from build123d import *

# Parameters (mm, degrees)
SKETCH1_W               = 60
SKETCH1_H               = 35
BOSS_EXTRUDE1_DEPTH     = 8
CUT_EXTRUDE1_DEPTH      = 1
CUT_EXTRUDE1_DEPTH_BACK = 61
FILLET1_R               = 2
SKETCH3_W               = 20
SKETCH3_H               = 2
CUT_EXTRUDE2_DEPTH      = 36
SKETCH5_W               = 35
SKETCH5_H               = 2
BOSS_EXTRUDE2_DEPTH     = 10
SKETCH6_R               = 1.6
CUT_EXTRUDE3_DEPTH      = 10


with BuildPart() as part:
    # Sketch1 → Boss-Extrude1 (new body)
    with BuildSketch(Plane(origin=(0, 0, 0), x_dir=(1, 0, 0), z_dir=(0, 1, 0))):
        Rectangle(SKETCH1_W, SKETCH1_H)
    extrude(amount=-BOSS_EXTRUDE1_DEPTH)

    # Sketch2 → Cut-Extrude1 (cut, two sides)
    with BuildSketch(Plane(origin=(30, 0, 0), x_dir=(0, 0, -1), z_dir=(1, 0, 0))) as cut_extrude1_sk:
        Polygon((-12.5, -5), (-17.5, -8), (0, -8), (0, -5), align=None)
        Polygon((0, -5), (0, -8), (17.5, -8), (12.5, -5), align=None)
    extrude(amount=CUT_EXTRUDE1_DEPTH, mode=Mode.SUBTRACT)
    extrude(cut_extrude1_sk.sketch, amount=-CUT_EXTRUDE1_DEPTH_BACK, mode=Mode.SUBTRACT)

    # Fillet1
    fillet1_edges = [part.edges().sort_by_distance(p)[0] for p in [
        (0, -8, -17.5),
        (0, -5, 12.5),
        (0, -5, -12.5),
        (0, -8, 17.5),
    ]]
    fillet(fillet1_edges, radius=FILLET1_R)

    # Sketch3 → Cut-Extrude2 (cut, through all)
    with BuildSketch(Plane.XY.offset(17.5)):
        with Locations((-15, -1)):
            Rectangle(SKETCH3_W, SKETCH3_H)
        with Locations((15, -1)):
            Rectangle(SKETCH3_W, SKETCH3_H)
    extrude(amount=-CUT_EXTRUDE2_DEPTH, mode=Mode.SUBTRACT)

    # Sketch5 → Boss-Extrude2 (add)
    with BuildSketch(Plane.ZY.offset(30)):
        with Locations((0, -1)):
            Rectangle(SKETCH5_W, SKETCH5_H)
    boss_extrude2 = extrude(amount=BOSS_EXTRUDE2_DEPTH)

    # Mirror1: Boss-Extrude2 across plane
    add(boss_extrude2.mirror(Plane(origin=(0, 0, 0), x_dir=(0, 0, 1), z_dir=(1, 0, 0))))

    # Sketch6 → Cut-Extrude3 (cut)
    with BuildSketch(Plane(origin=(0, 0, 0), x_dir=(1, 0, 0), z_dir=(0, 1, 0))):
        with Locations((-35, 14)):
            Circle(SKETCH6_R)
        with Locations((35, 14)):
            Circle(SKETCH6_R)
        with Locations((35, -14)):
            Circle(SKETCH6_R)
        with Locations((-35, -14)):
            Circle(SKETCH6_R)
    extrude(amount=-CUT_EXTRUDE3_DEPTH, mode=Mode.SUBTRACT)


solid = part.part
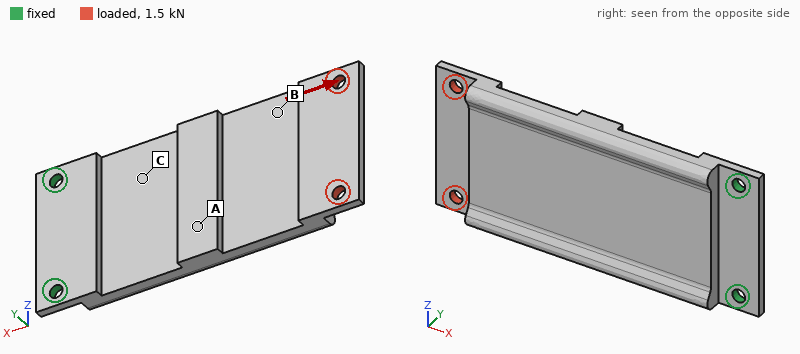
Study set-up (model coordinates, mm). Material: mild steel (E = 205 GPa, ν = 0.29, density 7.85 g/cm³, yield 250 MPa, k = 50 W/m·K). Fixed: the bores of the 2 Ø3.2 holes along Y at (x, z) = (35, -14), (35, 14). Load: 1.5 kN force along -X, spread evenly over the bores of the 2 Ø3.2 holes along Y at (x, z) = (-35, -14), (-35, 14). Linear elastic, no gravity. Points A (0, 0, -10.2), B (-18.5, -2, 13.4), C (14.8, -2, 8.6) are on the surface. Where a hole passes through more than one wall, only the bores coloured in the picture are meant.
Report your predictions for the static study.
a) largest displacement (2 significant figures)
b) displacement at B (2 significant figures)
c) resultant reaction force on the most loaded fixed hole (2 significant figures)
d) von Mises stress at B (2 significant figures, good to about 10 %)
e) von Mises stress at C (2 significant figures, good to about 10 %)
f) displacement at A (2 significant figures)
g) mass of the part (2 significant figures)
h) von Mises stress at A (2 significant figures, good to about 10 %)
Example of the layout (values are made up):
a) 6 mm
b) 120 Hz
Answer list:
a) 0.31 mm
b) 0.15 mm
c) 770 N
d) 73 MPa
e) 65 MPa
f) 0.060 mm
g) 75 g
h) 23 MPa
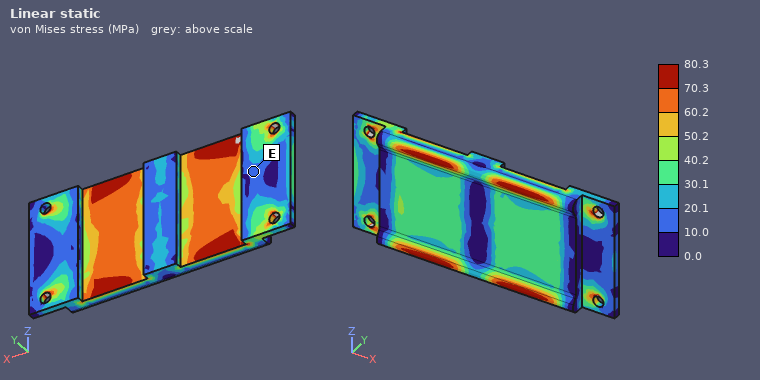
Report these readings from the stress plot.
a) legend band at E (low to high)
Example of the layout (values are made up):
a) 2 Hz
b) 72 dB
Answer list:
a) 10.0 to 20.1 MPa
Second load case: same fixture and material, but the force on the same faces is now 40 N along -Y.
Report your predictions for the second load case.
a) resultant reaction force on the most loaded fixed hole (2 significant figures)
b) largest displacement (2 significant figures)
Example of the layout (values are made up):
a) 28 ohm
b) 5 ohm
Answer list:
a) 53 N
b) 0.41 mm
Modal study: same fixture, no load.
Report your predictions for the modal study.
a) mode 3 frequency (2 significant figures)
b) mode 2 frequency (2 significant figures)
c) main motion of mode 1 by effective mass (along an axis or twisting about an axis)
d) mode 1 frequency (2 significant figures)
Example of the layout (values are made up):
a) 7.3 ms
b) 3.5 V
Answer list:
a) 2800 Hz
b) 2100 Hz
c) along Y
d) 350 Hz
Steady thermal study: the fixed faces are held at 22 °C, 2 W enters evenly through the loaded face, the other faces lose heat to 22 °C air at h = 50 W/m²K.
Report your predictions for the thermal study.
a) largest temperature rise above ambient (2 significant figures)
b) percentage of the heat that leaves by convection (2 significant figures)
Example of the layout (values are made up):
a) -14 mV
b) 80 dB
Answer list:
a) 15 K
b) 78 %
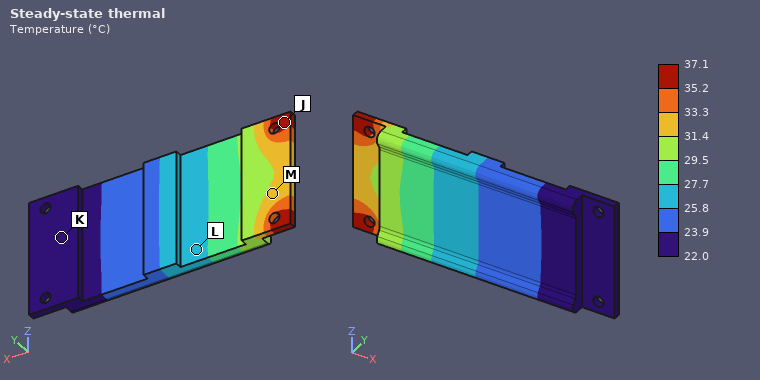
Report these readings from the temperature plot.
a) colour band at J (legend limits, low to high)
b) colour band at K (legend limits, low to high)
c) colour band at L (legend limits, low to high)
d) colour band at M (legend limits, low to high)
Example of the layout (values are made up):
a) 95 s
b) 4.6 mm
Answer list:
a) 35.2 to 37.1 °C
b) 22.0 to 23.9 °C
c) 25.8 to 27.7 °C
d) 31.4 to 33.3 °C
